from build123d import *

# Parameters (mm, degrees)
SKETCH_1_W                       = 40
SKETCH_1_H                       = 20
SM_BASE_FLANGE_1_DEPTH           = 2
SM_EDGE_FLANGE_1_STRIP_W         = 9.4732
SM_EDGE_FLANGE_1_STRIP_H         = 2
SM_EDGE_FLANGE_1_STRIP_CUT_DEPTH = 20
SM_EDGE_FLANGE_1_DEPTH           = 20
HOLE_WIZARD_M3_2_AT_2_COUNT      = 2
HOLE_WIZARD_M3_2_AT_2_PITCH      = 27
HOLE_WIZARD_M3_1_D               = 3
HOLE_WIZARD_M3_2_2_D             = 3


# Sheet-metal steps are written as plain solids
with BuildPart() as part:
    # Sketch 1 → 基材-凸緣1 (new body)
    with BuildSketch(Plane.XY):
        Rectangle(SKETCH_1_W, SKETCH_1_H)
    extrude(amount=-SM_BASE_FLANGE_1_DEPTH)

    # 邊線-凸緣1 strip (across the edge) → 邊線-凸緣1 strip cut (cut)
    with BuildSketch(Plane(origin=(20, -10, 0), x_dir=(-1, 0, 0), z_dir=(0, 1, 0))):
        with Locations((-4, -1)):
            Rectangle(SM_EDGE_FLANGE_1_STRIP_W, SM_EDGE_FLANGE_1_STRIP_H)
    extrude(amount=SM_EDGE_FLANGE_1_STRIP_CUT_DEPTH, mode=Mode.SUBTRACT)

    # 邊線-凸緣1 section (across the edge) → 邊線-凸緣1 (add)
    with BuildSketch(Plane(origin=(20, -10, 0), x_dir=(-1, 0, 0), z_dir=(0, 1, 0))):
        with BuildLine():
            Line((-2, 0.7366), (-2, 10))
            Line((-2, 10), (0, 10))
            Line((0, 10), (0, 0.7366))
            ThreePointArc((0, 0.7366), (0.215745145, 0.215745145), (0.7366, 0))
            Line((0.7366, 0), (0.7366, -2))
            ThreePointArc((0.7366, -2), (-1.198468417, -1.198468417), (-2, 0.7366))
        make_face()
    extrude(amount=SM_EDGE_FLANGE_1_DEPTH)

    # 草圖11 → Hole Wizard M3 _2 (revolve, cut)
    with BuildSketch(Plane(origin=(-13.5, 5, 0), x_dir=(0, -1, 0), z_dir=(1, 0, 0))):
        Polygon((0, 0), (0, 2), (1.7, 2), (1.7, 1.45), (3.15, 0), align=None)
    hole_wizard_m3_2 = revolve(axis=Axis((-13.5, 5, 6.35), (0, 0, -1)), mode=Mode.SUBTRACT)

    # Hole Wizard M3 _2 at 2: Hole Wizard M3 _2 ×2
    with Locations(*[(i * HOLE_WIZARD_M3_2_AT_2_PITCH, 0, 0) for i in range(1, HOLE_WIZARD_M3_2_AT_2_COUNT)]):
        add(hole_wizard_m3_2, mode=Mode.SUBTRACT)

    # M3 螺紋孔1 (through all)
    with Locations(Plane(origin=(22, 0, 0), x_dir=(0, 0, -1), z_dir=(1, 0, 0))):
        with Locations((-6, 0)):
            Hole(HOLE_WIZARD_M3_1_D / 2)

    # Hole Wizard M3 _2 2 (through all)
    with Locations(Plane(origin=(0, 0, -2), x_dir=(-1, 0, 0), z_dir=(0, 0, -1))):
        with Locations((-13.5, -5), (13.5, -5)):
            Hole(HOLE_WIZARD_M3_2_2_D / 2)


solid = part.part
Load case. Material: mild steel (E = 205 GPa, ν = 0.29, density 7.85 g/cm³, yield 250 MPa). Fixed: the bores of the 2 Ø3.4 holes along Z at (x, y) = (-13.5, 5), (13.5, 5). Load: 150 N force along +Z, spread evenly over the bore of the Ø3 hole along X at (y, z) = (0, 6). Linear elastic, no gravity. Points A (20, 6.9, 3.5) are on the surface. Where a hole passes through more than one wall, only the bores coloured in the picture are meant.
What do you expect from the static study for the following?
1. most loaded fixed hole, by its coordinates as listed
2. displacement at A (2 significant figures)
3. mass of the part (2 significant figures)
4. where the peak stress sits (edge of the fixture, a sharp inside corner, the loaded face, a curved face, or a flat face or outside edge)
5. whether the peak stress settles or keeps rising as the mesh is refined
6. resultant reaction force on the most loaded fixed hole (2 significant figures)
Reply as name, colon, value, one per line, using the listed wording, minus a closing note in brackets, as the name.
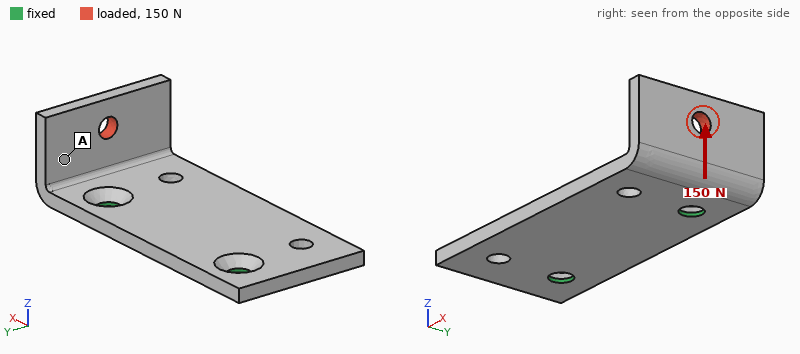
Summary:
most loaded fixed hole, by its coordinates as listed: (13.5, 5)
displacement at A: 22 µm
mass of the part: 15 g
where the peak stress sits: edge of the fixture
whether the peak stress settles or keeps rising as the mesh is refined: keeps rising
resultant reaction force on the most loaded fixed hole: 210 N
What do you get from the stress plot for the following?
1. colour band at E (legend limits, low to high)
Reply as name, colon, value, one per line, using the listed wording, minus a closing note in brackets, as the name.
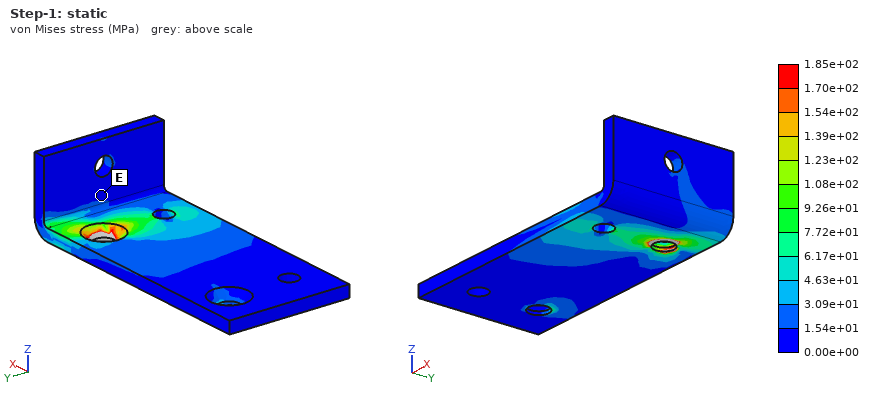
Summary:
colour band at E: 0.00e+00 to 1.54e+01 MPa
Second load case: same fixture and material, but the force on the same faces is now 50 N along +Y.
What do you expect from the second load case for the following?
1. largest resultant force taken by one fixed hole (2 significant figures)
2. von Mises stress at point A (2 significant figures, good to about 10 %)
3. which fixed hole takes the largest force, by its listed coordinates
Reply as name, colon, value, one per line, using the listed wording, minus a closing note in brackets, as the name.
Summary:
largest resultant force taken by one fixed hole: 60 N
von Mises stress at point A: 9.7 MPa
which fixed hole takes the largest force, by its listed coordinates: (13.5, 5)
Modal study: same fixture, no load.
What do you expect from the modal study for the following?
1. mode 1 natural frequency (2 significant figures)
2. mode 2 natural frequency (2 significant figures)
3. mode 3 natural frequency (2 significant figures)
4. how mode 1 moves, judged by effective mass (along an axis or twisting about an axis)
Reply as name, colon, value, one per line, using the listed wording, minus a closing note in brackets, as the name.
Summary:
mode 1 natural frequency: 3600 Hz
mode 2 natural frequency: 4700 Hz
mode 3 natural frequency: 6700 Hz
how mode 1 moves, judged by effective mass: along Z
